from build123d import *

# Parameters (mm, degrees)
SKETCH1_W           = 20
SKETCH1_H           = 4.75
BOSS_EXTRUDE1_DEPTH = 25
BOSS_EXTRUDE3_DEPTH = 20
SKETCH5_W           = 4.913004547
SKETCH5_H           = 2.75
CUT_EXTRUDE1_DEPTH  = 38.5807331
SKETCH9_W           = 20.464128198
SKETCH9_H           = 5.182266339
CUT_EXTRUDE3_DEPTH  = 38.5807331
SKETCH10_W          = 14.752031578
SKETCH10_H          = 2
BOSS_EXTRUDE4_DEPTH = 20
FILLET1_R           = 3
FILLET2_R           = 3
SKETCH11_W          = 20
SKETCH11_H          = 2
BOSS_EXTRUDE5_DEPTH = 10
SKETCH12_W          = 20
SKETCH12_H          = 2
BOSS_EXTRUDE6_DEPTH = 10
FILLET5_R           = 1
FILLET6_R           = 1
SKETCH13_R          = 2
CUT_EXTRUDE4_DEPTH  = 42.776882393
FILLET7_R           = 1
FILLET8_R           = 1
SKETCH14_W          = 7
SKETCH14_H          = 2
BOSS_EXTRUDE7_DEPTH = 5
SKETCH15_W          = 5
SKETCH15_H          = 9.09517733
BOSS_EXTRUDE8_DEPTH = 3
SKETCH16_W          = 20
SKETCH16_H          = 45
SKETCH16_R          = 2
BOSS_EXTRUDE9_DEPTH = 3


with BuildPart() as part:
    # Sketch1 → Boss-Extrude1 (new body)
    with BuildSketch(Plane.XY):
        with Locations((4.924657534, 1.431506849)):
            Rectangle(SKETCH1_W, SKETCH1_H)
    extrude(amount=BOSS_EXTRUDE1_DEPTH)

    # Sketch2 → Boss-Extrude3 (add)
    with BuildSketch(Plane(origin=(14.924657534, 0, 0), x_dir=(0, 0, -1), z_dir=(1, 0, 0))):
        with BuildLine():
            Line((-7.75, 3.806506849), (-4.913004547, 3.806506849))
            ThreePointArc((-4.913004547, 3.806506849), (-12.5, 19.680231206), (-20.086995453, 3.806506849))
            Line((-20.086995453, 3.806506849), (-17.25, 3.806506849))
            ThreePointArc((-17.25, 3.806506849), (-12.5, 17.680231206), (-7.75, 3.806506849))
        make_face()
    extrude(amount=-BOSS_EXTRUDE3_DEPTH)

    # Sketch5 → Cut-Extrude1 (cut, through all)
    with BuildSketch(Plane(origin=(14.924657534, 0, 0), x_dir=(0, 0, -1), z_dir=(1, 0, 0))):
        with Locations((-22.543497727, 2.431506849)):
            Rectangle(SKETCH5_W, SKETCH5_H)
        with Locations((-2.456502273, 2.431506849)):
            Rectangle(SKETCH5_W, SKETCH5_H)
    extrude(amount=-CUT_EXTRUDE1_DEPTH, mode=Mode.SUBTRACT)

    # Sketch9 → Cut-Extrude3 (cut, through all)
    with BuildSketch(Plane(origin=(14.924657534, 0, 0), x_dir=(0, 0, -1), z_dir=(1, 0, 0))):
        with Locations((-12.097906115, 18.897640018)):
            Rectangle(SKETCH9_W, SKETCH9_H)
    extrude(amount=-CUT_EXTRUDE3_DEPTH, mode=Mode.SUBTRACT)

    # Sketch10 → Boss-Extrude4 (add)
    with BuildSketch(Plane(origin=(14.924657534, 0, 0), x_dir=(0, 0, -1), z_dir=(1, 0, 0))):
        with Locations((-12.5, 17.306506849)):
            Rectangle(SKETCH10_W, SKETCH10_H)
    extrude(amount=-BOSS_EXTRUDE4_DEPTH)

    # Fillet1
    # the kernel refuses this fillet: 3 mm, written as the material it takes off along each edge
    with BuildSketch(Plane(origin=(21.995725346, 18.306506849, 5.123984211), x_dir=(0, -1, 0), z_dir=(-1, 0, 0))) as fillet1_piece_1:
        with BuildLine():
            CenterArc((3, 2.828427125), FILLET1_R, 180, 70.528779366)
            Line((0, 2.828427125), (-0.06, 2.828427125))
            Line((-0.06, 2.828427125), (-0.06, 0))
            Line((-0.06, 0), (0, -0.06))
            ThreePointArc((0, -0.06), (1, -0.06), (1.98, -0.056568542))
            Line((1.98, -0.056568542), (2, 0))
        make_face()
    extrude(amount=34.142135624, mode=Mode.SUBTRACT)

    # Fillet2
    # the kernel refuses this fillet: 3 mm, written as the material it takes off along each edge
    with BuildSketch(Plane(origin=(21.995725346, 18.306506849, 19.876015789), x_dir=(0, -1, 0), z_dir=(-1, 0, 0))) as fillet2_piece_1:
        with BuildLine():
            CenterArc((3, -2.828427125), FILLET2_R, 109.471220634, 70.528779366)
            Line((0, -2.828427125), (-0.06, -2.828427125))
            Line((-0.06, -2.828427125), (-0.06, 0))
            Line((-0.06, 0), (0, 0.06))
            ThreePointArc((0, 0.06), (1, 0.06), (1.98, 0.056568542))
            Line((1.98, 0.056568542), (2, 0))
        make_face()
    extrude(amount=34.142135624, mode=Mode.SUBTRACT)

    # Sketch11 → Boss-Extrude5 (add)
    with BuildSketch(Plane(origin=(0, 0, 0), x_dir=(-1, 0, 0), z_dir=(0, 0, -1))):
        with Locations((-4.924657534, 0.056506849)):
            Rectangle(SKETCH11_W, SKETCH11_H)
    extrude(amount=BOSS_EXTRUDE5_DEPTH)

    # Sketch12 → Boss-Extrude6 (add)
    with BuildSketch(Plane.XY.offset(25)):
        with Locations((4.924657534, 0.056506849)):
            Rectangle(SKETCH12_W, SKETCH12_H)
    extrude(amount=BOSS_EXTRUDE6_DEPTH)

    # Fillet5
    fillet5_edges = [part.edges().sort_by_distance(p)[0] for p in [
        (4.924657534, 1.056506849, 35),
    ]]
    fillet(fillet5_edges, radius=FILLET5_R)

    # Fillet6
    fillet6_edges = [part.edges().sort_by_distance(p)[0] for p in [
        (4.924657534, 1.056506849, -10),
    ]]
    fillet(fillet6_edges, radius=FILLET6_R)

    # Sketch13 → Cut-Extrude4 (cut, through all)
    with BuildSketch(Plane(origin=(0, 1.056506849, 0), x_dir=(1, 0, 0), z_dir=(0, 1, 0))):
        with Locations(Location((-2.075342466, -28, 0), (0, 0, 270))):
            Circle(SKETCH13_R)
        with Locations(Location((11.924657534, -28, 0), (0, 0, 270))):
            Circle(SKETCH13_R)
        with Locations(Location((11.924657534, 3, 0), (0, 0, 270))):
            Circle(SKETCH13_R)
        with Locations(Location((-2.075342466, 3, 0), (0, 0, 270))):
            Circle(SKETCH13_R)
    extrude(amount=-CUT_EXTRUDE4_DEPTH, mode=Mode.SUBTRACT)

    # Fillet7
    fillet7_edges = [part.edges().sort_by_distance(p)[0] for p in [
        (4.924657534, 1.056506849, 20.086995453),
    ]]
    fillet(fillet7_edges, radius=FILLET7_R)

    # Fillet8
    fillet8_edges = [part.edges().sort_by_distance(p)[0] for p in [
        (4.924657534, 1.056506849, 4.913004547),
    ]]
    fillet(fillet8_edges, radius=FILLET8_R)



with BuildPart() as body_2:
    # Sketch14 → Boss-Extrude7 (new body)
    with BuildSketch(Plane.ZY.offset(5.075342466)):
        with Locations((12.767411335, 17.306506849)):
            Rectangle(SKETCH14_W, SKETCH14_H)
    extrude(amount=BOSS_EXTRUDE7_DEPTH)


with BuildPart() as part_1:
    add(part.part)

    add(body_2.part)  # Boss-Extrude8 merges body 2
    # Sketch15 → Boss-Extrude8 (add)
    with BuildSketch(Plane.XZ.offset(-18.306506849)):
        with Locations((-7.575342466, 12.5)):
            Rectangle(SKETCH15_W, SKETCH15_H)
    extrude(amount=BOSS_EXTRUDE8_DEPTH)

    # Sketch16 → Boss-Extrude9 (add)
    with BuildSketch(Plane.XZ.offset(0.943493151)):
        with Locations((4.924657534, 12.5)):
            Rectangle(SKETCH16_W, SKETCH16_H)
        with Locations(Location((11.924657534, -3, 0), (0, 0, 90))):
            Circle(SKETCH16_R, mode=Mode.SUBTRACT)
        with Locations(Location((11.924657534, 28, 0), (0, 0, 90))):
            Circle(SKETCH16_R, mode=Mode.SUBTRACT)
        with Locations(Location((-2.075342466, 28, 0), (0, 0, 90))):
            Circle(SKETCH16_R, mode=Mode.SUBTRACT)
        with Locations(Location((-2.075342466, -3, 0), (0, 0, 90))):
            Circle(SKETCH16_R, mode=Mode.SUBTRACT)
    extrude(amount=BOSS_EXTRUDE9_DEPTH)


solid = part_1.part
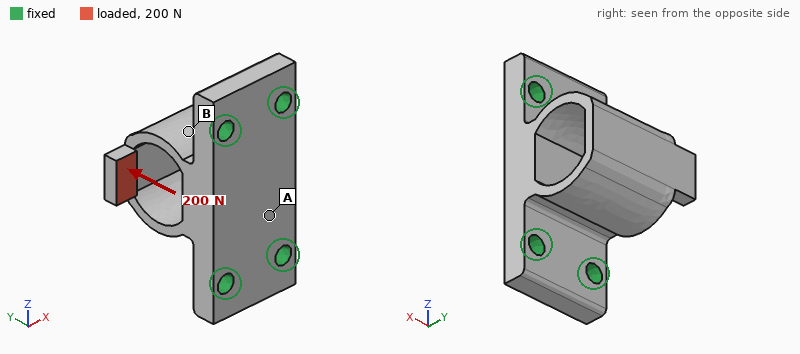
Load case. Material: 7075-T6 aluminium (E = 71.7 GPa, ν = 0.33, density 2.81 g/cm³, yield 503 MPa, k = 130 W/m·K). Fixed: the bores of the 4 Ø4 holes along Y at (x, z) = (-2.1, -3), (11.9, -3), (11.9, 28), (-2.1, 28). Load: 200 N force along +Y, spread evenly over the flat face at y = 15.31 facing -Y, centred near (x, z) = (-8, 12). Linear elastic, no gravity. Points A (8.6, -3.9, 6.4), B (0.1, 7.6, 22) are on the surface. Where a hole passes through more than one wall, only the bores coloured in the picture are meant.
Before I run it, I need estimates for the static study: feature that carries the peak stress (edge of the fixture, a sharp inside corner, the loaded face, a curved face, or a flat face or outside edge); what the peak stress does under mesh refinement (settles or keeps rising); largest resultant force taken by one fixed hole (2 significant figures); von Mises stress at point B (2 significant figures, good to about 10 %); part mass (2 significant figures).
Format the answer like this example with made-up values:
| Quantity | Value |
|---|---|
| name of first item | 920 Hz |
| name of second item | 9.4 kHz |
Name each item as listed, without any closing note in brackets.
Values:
| Quantity | Value |
|---|---|
| feature that carries the peak stress | a sharp inside corner |
| what the peak stress does under mesh refinement | keeps rising |
| largest resultant force taken by one fixed hole | 130 N |
| von Mises stress at point B | 15 MPa |
| part mass | 19 g |
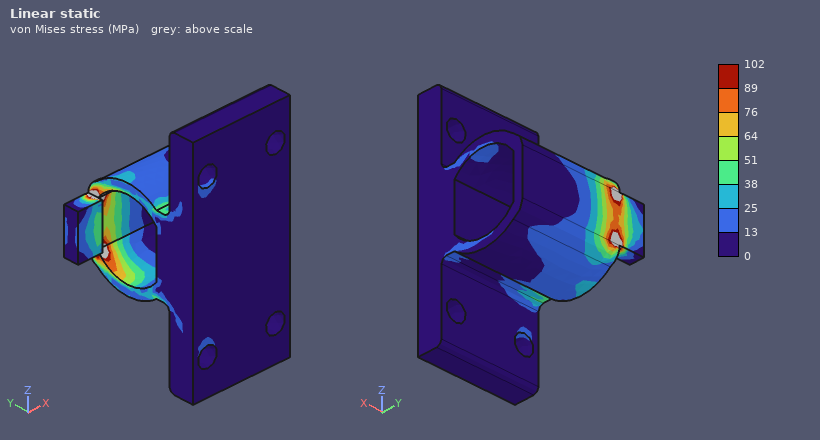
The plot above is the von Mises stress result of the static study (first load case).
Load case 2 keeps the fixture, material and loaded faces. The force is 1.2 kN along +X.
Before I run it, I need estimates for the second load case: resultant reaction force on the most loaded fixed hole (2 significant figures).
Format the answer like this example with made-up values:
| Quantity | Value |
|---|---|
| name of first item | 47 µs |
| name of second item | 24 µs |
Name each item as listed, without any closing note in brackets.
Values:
| Quantity | Value |
|---|---|
| resultant reaction force on the most loaded fixed hole | 800 N |
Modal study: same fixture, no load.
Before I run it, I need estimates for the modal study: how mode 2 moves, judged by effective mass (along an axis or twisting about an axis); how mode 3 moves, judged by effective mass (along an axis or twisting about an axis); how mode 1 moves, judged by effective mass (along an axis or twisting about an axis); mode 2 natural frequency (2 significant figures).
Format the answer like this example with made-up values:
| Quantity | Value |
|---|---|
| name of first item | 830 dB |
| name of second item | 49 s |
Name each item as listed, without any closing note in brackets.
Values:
| Quantity | Value |
|---|---|
| how mode 2 moves, judged by effective mass | along X |
| how mode 3 moves, judged by effective mass | along Y |
| how mode 1 moves, judged by effective mass | along Z |
| mode 2 natural frequency | 11 kHz |
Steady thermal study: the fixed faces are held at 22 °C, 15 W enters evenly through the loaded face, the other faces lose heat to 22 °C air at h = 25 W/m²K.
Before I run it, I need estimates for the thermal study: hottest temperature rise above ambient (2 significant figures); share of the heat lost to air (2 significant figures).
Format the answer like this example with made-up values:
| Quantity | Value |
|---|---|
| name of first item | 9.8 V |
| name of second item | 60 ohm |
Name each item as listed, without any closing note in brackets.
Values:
| Quantity | Value |
|---|---|
| hottest temperature rise above ambient | 68 K |
| share of the heat lost to air | 8.0 % |
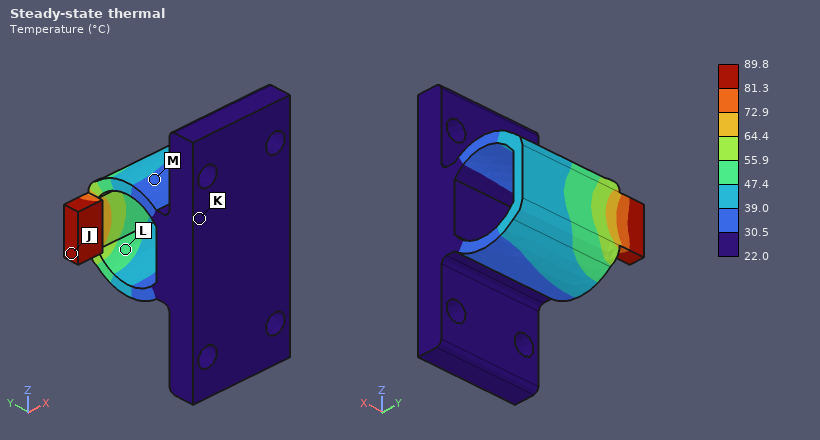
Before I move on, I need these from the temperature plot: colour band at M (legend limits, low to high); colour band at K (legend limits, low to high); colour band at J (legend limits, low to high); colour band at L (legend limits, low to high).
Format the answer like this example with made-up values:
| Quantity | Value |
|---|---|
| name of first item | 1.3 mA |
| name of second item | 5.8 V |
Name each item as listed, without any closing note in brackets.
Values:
| Quantity | Value |
|---|---|
| colour band at M | 30.5 to 39.0 °C |
| colour band at K | 22.0 to 30.5 °C |
| colour band at J | 81.3 to 89.8 °C |
| colour band at L | 47.4 to 55.9 °C |
